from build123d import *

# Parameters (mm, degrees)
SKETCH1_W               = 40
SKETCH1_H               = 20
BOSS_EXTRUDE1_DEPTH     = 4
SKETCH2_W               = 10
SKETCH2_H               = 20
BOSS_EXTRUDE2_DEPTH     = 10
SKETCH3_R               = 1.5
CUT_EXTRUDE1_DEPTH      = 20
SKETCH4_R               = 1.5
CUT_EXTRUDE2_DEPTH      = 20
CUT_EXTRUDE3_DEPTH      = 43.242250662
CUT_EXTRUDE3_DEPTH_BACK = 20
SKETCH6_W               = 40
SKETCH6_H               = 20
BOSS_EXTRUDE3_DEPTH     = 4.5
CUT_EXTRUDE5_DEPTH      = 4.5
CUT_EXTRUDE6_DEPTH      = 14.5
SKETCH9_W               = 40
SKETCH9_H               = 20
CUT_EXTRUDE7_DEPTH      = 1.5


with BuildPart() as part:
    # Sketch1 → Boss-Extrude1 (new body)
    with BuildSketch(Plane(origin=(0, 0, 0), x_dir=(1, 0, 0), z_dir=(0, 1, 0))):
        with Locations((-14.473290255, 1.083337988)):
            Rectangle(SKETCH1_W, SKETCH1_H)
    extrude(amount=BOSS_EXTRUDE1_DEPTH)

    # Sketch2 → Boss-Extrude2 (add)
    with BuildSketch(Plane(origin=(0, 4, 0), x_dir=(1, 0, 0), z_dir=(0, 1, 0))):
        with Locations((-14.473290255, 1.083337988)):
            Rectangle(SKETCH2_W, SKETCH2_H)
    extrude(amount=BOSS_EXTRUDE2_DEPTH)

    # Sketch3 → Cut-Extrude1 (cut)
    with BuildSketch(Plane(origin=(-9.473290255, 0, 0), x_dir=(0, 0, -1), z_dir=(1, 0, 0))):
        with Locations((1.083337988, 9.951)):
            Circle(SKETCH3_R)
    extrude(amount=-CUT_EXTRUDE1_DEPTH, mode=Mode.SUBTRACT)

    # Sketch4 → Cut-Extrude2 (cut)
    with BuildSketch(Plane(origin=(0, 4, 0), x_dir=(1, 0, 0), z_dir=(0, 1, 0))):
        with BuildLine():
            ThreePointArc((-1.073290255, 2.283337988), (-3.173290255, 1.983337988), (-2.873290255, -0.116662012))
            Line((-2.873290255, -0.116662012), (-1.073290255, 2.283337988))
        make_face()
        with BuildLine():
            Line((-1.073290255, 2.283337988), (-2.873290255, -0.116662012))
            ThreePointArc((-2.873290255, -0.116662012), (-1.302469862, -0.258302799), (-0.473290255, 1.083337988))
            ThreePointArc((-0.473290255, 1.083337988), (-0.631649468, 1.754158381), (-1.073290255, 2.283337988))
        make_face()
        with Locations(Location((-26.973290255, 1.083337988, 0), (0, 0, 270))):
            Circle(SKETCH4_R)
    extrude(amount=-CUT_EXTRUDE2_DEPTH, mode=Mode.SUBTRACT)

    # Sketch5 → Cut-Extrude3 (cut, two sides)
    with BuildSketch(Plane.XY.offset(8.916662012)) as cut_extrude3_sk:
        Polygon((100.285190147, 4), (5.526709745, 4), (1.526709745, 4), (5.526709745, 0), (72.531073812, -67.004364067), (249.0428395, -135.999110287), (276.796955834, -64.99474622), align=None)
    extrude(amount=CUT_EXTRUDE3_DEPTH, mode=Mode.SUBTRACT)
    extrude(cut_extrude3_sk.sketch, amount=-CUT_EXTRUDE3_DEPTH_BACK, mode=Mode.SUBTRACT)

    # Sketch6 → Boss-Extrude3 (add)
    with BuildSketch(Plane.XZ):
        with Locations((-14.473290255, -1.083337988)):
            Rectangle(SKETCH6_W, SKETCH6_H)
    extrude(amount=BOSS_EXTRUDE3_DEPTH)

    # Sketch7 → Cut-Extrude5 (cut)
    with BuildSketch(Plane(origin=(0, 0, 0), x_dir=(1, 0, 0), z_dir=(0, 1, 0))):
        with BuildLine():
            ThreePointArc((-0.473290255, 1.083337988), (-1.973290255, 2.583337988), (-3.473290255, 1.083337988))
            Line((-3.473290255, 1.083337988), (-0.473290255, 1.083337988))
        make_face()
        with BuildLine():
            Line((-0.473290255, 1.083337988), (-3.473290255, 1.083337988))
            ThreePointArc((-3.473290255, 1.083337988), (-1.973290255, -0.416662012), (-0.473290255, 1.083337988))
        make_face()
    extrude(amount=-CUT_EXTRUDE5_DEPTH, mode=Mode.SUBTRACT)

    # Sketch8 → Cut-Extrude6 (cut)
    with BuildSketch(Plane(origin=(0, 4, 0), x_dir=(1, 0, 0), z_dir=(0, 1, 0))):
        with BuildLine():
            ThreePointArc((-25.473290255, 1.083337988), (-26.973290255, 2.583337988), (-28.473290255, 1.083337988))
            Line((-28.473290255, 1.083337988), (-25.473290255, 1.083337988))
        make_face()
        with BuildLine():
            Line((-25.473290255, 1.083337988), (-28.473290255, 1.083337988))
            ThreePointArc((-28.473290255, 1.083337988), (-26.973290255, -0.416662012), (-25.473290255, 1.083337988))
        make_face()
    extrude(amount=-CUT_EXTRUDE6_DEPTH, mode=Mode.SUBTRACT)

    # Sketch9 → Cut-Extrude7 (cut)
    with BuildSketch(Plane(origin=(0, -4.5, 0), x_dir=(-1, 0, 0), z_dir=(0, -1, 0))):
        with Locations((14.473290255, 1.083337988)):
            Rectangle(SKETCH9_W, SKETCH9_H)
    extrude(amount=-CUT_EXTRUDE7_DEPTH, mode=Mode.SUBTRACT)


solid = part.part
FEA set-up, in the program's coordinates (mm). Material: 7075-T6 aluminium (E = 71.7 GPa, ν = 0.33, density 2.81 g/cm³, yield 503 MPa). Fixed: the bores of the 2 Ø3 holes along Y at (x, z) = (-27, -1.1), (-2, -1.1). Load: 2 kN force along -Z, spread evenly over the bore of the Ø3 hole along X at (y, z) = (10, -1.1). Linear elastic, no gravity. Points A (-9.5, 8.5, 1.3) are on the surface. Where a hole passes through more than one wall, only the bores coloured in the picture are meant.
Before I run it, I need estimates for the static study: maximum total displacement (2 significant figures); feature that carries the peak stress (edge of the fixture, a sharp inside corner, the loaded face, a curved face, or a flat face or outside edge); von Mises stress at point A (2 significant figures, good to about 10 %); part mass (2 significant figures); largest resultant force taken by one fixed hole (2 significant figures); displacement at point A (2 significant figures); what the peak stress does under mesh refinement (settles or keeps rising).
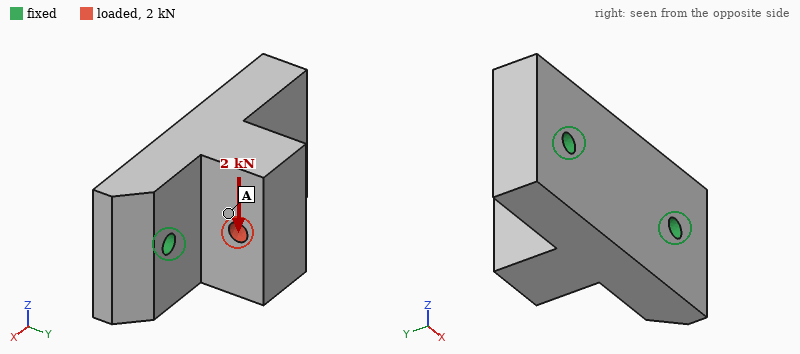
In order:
40 µm
edge of the fixture
24 MPa
20 g
1.0 kN
23 µm
keeps rising
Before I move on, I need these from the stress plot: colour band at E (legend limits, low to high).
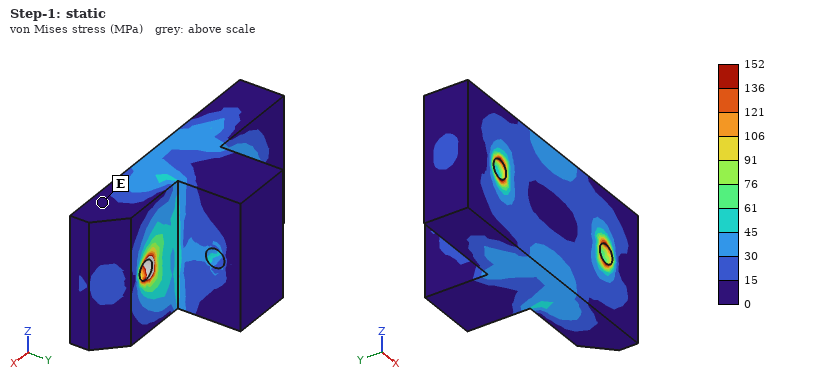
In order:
0 to 15 MPa
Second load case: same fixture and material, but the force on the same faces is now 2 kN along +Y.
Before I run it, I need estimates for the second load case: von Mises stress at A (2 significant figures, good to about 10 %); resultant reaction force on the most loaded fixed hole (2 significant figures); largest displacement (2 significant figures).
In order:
23 MPa
1.0 kN
9.8 µm
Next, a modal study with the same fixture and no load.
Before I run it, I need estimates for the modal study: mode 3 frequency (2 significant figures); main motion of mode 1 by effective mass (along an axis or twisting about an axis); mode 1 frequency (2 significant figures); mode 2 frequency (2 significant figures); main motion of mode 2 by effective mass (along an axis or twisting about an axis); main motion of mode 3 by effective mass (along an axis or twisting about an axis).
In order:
28 kHz
along Z
16 kHz
25 kHz
along Y
along X
